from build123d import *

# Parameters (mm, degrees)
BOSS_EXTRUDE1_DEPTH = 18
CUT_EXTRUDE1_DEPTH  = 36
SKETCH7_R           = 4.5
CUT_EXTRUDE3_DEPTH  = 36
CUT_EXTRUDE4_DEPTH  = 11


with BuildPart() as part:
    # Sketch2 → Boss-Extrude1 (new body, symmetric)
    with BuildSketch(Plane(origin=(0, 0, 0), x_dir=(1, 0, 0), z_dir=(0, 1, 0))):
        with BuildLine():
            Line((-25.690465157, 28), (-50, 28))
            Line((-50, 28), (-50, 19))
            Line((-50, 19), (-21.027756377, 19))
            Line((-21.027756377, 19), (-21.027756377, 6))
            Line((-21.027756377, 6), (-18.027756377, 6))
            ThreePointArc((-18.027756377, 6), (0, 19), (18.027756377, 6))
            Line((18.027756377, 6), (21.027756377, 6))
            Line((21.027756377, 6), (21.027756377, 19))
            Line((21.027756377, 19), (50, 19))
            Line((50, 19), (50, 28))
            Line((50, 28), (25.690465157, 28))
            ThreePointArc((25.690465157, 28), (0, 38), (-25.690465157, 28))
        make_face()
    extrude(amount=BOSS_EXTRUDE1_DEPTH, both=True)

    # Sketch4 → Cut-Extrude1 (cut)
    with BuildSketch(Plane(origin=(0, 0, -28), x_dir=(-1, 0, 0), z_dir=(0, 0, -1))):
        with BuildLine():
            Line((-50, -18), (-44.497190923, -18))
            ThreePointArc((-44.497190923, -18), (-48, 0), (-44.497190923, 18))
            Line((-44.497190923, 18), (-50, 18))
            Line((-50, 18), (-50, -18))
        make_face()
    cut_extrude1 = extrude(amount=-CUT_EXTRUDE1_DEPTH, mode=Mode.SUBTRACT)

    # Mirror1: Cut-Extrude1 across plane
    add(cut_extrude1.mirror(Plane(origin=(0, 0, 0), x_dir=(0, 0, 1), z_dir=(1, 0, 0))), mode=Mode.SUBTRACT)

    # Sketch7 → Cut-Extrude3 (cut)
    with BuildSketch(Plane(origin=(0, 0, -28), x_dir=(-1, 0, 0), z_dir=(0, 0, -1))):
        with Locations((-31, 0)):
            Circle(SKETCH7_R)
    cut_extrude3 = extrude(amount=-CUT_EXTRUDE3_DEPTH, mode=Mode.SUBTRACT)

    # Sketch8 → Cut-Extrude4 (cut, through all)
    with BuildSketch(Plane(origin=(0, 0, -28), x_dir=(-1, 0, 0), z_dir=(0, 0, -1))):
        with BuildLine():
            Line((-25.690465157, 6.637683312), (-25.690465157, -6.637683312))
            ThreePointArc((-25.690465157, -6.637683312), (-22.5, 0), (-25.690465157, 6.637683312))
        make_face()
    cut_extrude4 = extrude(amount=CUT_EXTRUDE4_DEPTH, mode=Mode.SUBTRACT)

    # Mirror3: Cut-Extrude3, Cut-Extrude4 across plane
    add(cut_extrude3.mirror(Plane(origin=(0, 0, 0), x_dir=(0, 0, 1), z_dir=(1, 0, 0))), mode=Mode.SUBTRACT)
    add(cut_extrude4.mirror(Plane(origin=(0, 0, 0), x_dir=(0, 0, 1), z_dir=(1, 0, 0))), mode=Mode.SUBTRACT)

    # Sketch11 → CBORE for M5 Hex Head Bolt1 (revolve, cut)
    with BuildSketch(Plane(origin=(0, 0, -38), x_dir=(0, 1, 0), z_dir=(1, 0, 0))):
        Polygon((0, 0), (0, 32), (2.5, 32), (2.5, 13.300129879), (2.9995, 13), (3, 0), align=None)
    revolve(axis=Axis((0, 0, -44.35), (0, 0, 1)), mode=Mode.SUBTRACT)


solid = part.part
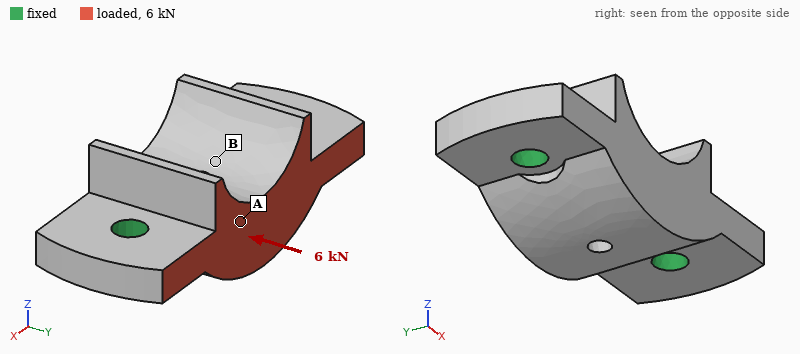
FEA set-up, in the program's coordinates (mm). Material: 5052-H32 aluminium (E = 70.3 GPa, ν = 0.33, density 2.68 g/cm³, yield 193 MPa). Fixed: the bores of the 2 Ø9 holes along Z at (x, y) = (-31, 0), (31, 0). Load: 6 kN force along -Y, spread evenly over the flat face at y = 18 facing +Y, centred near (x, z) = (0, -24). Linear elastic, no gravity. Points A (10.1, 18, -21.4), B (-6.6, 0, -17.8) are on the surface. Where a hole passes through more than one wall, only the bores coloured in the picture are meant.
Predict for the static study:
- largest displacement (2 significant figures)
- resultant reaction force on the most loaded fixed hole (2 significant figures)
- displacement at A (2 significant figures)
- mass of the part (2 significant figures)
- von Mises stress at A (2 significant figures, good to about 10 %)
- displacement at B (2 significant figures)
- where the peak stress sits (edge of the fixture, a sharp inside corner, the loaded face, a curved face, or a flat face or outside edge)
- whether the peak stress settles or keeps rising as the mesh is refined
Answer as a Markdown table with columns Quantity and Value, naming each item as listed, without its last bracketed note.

| Quantity | Value |
|---|---|
| largest displacement | 9.4 µm |
| resultant reaction force on the most loaded fixed hole | 3.0 kN |
| displacement at A | 6.1 µm |
| mass of the part | 130 g |
| von Mises stress at A | 9.4 MPa |
| displacement at B | 4.9 µm |
| where the peak stress sits | edge of the fixture |
| whether the peak stress settles or keeps rising as the mesh is refined | keeps rising |
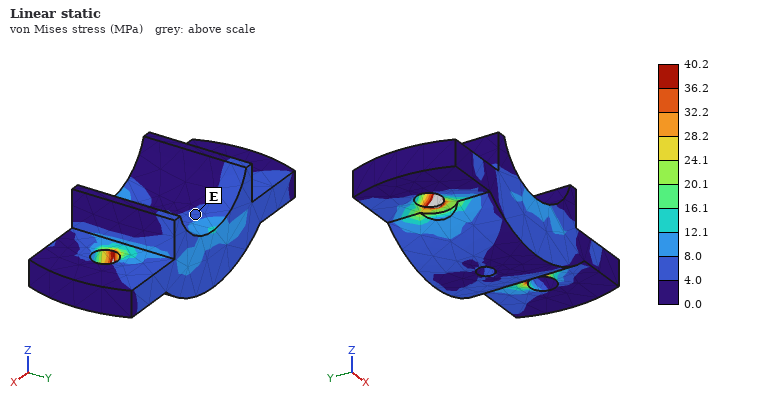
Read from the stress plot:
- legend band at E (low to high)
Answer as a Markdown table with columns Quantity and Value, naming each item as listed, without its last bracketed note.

| Quantity | Value |
|---|---|
| legend band at E | 4.0 to 8.0 MPa |
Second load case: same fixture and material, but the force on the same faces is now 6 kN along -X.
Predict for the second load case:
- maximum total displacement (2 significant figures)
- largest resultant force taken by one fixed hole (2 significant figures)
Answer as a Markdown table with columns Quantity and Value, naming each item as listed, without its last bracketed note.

| Quantity | Value |
|---|---|
| maximum total displacement | 11 µm |
| largest resultant force taken by one fixed hole | 3.4 kN |
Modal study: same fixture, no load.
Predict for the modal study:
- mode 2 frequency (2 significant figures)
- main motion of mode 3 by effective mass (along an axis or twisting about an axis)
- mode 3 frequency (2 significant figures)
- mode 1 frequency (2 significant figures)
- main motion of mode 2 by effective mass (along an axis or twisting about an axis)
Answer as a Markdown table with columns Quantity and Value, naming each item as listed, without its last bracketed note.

| Quantity | Value |
|---|---|
| mode 2 frequency | 12 kHz |
| main motion of mode 3 by effective mass | along Y |
| mode 3 frequency | 15 kHz |
| mode 1 frequency | 9100 Hz |
| main motion of mode 2 by effective mass | along Z |
